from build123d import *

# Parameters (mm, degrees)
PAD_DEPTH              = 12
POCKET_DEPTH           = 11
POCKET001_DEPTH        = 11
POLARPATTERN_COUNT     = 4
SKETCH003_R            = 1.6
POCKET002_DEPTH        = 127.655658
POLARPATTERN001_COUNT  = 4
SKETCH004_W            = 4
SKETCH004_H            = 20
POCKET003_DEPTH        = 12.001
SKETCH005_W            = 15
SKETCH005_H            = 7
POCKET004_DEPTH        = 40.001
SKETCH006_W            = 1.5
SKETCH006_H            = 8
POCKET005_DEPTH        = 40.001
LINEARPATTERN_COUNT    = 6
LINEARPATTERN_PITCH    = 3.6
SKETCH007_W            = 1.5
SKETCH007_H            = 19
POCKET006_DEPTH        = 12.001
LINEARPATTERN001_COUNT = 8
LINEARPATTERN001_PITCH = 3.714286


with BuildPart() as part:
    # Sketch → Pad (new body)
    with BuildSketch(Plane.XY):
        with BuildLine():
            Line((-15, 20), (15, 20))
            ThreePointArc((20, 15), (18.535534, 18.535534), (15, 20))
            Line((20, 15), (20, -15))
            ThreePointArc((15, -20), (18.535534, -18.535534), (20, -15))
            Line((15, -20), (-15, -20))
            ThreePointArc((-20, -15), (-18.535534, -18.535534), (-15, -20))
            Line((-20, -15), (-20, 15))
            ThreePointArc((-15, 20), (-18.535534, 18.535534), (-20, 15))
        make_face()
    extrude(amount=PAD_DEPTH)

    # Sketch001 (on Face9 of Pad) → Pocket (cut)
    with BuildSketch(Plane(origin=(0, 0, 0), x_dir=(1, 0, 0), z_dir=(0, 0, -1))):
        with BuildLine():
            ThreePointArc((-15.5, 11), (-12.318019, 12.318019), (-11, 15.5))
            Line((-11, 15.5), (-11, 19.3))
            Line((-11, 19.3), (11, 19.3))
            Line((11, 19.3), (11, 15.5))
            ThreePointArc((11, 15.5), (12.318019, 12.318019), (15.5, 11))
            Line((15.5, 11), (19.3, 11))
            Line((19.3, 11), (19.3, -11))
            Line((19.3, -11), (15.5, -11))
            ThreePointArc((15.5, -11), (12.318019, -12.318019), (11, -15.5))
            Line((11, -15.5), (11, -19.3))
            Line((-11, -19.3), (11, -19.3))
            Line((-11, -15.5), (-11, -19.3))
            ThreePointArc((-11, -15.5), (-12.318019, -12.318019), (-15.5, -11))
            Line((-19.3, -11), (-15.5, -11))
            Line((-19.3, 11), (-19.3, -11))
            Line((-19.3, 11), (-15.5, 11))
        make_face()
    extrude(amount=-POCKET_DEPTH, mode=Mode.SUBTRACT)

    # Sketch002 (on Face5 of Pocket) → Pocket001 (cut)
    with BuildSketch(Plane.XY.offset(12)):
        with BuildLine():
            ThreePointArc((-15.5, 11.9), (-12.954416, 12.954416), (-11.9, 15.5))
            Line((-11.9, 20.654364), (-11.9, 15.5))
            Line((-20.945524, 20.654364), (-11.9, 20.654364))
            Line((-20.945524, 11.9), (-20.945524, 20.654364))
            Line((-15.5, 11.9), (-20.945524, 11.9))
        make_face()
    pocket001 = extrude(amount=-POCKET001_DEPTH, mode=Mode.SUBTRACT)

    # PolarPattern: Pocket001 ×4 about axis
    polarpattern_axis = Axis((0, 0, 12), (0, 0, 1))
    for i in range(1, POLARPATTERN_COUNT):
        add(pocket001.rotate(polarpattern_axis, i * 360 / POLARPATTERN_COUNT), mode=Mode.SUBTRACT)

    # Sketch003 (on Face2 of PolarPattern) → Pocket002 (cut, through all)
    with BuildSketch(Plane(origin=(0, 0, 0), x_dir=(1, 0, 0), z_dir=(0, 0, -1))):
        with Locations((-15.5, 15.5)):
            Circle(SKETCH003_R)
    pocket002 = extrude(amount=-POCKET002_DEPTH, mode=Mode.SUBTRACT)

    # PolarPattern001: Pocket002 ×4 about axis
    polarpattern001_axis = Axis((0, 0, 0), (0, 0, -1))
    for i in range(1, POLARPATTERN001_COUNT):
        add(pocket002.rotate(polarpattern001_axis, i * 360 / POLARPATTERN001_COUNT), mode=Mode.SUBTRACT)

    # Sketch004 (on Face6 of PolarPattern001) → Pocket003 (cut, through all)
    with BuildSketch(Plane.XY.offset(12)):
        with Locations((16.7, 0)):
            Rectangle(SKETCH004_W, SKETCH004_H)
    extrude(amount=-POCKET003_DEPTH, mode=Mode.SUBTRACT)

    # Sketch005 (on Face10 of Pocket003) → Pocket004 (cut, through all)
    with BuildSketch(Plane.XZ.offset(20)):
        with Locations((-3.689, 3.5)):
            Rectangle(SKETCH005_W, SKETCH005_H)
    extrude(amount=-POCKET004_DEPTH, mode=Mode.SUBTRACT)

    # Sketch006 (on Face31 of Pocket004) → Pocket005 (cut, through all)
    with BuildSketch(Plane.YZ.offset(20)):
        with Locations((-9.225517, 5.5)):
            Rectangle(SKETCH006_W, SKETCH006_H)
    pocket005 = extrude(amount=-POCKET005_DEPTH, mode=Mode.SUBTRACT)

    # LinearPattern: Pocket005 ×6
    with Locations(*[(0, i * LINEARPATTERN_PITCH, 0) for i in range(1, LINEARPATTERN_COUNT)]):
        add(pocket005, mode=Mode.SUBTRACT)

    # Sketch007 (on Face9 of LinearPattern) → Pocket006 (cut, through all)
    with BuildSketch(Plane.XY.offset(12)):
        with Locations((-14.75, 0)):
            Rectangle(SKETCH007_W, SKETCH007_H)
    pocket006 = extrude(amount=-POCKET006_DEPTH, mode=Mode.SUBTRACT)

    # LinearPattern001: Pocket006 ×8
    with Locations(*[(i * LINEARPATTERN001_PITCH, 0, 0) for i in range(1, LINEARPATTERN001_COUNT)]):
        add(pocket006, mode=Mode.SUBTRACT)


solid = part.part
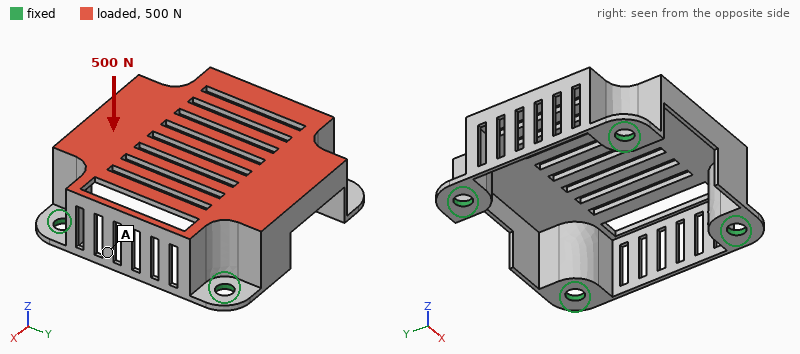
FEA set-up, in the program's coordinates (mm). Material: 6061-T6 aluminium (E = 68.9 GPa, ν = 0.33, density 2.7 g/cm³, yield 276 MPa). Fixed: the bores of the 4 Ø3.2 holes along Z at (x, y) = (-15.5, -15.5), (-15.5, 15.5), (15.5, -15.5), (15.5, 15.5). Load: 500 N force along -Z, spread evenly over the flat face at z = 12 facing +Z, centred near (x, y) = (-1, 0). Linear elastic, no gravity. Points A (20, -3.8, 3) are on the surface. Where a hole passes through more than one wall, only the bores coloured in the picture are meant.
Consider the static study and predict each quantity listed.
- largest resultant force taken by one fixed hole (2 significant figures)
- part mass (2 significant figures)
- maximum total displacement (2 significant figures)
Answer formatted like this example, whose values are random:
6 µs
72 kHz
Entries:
140 N
6.1 g
0.33 mm
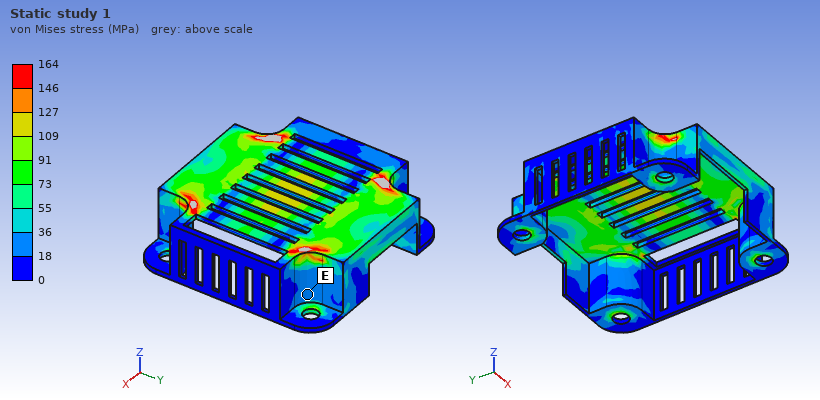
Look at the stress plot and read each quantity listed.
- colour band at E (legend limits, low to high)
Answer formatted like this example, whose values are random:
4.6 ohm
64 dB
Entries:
18 to 36 MPa
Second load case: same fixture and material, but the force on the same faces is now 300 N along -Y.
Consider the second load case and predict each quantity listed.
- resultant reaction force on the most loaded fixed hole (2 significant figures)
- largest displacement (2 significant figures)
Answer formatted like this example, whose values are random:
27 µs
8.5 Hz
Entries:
100 N
45 µm
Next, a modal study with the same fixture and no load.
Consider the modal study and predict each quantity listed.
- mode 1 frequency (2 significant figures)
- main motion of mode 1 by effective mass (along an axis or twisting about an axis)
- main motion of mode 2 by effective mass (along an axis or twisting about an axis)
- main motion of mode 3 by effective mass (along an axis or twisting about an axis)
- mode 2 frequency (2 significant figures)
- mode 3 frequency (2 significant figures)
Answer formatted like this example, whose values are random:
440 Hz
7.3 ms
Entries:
4900 Hz
along Z
along X
along X
6300 Hz
7000 Hz
